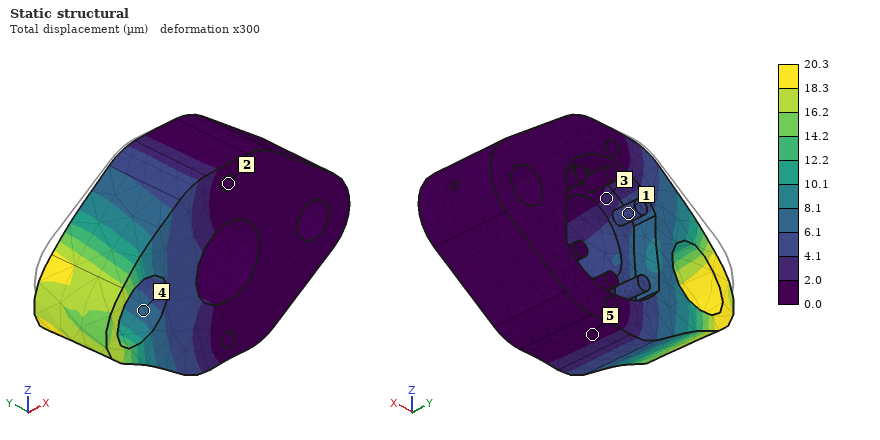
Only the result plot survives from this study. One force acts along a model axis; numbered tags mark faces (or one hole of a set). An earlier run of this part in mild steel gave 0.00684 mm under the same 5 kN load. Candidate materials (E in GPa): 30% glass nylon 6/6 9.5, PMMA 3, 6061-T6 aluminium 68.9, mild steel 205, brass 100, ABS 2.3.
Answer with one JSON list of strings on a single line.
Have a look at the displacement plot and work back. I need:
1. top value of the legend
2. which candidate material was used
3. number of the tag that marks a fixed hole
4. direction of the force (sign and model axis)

["20.3 µm", "6061-T6 aluminium", "2", "-Z"]
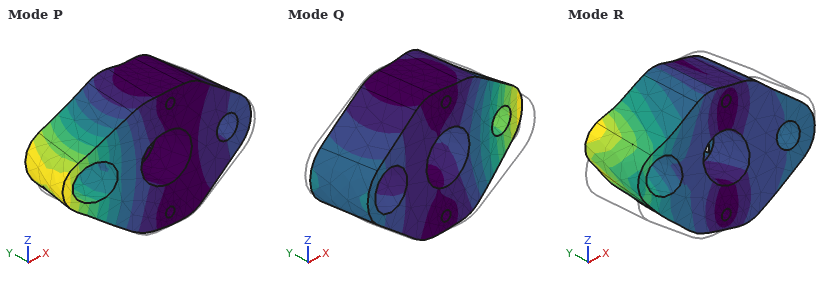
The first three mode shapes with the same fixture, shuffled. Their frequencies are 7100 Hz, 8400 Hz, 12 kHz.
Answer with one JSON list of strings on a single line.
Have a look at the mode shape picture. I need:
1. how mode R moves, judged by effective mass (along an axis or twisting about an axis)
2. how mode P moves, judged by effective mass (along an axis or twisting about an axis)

["twisting about Y", "along Y"]
